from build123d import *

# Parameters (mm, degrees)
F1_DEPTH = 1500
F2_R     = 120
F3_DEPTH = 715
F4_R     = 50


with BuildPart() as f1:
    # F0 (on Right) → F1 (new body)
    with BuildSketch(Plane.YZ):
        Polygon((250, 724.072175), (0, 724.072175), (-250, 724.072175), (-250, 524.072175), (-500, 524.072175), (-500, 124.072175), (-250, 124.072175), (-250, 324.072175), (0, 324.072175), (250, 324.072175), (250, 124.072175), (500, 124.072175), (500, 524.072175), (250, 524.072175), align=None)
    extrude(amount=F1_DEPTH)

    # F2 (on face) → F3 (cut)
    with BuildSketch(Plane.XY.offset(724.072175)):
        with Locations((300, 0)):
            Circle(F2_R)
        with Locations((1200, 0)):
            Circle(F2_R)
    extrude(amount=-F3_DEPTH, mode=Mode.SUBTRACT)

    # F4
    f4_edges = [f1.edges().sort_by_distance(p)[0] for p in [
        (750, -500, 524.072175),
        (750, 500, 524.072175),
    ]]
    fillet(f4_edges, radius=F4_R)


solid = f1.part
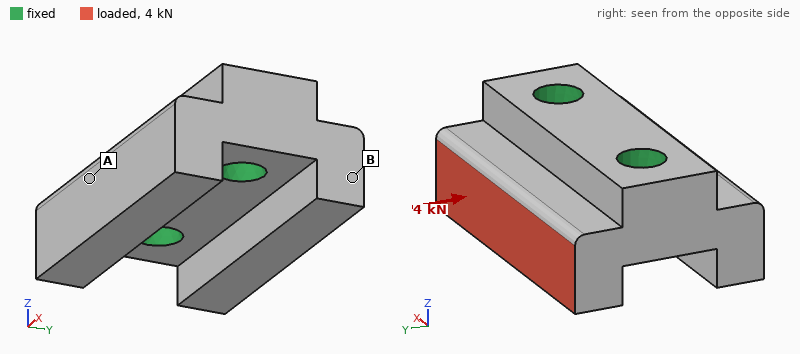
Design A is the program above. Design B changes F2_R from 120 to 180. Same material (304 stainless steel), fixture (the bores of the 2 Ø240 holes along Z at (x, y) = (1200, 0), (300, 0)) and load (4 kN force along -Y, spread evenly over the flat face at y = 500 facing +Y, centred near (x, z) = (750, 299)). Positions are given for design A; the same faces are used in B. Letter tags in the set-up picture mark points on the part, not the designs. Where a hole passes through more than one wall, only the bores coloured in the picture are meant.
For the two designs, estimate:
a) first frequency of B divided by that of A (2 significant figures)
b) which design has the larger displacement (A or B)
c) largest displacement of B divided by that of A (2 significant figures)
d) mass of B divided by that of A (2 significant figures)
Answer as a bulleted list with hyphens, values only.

- 1.2
- A
- 0.83
- 0.92
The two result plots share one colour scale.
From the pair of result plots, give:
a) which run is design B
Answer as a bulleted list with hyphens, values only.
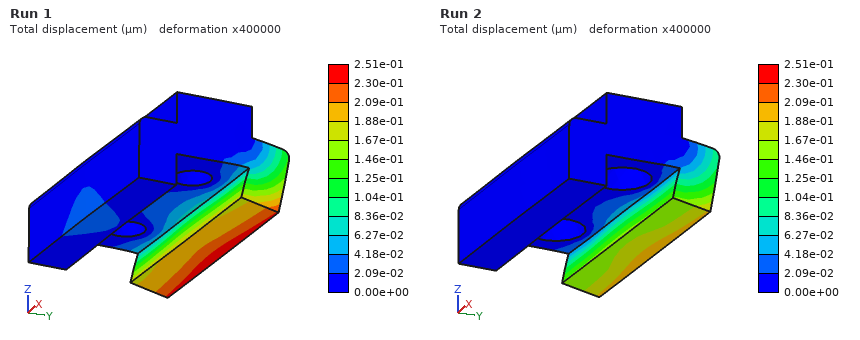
- Run 2
